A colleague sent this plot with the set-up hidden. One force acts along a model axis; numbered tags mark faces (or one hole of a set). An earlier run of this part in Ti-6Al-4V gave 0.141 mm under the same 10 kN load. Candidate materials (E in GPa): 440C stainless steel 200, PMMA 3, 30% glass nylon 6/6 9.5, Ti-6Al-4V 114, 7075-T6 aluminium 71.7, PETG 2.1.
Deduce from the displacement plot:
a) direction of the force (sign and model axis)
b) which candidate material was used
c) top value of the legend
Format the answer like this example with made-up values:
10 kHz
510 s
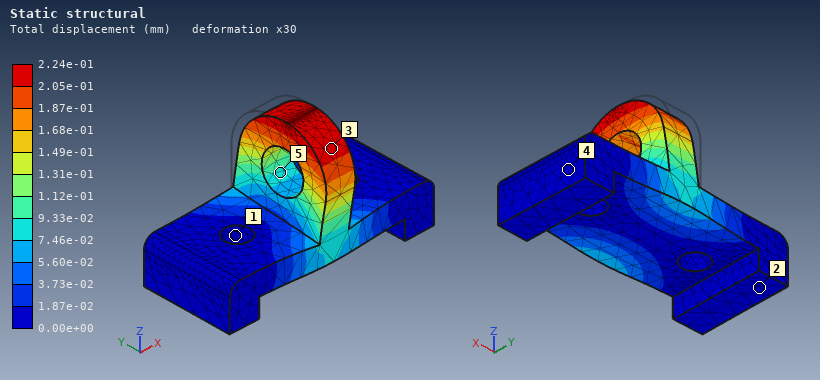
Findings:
-Y
7075-T6 aluminium
2.24e-01 mm
